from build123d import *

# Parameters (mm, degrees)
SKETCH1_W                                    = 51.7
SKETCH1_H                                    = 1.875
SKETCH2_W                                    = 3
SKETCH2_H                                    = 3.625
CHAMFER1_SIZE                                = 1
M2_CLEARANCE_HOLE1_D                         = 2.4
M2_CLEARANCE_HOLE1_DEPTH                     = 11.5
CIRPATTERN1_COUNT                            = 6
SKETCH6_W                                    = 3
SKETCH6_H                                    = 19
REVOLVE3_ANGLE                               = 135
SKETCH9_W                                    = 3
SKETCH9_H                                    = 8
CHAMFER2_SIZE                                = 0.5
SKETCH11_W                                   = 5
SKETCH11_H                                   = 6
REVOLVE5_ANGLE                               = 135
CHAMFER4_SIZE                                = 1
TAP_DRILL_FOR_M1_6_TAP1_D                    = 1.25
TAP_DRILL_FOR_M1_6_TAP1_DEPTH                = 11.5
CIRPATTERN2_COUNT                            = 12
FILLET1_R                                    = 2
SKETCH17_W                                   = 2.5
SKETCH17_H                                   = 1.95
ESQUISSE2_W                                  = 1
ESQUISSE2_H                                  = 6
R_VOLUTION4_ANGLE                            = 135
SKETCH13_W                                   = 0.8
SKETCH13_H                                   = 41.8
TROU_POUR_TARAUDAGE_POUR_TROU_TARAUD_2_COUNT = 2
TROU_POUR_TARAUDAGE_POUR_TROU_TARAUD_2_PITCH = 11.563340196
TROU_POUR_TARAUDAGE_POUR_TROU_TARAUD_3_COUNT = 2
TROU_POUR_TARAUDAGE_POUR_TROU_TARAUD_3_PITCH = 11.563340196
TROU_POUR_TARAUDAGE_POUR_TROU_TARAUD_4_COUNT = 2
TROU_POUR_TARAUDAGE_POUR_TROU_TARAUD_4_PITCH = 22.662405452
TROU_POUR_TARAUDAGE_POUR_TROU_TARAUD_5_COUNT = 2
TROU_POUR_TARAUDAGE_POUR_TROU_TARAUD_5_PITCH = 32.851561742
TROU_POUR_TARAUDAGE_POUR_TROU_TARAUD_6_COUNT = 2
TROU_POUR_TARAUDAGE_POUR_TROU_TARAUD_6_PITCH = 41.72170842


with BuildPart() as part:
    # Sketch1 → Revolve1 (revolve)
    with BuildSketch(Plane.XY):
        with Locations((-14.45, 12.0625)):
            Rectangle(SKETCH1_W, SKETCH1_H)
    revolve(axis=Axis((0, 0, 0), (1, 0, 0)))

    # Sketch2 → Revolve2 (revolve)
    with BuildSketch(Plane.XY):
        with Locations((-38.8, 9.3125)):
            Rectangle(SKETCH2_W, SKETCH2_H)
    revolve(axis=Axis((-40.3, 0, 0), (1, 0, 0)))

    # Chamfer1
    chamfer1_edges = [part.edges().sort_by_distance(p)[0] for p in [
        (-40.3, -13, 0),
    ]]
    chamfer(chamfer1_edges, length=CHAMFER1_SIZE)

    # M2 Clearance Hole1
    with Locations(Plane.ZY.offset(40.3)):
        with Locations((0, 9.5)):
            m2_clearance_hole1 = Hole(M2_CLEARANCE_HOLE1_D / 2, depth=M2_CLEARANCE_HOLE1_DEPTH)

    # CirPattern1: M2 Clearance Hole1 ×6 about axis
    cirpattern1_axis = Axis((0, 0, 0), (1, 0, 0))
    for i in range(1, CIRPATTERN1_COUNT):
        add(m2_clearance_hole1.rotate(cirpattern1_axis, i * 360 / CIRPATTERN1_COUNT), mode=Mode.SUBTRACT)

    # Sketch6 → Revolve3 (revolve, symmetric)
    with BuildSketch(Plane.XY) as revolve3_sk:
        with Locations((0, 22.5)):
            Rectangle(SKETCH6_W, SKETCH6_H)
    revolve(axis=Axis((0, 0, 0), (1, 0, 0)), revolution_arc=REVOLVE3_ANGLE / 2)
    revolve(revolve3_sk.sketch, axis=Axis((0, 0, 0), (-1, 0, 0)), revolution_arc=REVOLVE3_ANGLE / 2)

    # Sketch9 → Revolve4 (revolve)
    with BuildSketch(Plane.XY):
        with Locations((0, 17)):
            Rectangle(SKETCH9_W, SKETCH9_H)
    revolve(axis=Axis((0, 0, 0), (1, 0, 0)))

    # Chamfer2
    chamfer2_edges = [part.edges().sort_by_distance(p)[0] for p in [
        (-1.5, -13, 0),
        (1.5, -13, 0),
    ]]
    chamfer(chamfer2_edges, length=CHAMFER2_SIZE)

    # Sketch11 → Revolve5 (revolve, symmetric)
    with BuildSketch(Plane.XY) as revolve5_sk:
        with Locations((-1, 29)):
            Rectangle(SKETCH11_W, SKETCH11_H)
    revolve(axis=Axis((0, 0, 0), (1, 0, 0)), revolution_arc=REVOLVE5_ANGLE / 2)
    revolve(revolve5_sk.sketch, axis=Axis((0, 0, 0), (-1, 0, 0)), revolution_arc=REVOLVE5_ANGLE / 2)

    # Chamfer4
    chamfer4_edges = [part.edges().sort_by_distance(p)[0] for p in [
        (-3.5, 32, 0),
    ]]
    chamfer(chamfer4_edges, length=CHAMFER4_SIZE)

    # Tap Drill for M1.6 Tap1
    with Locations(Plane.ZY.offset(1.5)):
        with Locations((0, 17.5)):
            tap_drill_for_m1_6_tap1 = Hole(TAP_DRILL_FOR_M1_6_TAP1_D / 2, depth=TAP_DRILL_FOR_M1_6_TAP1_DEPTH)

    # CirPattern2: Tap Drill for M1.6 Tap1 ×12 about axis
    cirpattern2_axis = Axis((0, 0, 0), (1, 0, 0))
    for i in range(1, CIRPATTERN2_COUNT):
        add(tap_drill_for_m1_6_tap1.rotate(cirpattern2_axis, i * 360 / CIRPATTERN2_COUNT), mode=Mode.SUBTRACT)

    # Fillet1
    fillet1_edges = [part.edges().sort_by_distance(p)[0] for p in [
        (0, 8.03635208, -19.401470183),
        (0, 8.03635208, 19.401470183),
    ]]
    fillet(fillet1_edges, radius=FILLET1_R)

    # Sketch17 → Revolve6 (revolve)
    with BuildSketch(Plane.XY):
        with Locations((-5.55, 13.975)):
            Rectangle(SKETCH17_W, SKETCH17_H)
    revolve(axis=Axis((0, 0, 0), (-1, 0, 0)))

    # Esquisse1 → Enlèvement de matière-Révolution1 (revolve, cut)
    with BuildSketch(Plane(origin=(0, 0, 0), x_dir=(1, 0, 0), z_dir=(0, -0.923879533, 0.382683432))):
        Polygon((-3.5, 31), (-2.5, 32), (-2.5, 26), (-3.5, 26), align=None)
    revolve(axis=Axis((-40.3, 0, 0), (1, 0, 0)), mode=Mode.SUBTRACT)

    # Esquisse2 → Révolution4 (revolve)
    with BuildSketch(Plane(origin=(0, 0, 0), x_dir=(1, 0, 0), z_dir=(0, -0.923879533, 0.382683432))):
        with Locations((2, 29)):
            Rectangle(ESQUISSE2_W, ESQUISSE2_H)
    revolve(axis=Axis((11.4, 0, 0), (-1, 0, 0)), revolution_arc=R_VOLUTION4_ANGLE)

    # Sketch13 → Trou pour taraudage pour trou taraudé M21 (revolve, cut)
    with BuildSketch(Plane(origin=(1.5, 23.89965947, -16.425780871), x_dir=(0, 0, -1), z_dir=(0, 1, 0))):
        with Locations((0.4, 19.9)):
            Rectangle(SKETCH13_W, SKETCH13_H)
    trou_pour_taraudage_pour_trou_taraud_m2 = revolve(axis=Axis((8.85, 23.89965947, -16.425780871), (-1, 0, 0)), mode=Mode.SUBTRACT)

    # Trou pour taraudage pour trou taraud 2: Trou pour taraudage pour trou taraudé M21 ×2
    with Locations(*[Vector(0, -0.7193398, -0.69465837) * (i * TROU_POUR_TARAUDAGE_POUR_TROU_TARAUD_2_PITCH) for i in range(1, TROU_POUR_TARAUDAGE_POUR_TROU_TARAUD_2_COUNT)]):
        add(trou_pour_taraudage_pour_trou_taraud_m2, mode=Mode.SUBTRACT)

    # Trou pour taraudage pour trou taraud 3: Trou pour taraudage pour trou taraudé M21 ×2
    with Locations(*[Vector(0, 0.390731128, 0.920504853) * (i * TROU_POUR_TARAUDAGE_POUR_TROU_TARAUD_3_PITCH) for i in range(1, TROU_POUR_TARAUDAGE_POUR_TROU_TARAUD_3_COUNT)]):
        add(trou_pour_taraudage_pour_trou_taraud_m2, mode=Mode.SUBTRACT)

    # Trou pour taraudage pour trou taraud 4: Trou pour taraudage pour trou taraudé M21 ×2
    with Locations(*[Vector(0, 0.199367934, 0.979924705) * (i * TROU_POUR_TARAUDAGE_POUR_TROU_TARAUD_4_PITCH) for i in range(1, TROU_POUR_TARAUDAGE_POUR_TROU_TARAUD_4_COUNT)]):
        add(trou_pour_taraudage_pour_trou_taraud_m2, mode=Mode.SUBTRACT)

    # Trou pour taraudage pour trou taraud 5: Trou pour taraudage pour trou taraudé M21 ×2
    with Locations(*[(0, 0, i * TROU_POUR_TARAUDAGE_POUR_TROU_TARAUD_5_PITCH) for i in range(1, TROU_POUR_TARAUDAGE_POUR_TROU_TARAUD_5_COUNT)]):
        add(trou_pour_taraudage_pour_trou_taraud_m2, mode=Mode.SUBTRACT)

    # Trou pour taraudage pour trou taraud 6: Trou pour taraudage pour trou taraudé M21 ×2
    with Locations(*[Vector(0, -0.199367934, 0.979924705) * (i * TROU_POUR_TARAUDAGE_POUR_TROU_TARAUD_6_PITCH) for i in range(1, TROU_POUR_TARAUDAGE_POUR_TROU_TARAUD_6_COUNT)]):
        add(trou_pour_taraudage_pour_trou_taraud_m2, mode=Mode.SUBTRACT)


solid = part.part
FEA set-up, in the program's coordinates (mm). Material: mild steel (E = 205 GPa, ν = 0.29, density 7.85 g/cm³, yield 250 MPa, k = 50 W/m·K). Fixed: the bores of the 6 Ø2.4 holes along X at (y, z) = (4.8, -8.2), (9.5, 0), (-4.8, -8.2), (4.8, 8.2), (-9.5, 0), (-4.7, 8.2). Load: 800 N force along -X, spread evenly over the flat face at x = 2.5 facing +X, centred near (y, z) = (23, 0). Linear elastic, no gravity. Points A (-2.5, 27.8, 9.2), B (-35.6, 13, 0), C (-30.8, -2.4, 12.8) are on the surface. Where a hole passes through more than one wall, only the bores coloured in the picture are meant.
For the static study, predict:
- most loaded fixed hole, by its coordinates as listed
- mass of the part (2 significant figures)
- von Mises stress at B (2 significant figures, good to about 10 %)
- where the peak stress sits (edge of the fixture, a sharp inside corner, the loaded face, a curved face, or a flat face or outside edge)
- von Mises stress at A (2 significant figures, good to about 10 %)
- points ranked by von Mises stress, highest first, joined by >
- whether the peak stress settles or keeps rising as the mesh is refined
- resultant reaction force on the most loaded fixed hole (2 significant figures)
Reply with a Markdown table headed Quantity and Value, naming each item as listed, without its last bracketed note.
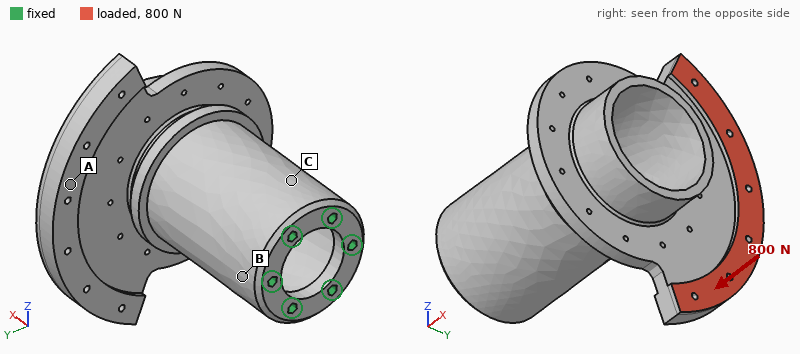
| Quantity | Value |
|---|---|
| most loaded fixed hole, by its coordinates as listed | (9.5, 0) |
| mass of the part | 110 g |
| von Mises stress at B | 30 MPa |
| where the peak stress sits | edge of the fixture |
| von Mises stress at A | 39 MPa |
| points ranked by von Mises stress, highest first, joined by > | A > B > C |
| whether the peak stress settles or keeps rising as the mesh is refined | keeps rising |
| resultant reaction force on the most loaded fixed hole | 610 N |
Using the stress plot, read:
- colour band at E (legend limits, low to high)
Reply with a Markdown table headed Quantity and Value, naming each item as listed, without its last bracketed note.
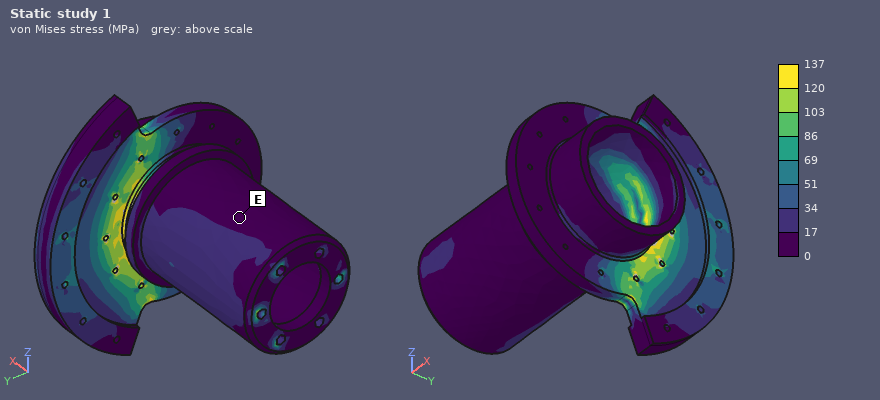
| Quantity | Value |
|---|---|
| colour band at E | 0 to 17 MPa |
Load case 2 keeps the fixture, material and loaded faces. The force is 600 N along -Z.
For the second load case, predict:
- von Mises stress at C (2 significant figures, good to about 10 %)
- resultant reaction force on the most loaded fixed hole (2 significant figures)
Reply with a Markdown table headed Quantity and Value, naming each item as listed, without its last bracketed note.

| Quantity | Value |
|---|---|
| von Mises stress at C | 27 MPa |
| resultant reaction force on the most loaded fixed hole | 680 N |
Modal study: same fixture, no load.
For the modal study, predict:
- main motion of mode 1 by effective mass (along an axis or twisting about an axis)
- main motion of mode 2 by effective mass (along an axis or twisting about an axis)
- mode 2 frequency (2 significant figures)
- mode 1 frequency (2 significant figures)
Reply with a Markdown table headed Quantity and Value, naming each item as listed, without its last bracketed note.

| Quantity | Value |
|---|---|
| main motion of mode 1 by effective mass | along Y |
| main motion of mode 2 by effective mass | along Z |
| mode 2 frequency | 3500 Hz |
| mode 1 frequency | 3300 Hz |
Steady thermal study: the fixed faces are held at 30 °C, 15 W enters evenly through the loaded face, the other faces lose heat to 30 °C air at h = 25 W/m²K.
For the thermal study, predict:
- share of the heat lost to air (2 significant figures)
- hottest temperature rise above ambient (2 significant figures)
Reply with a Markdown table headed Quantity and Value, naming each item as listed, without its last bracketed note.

| Quantity | Value |
|---|---|
| share of the heat lost to air | 61 % |
| hottest temperature rise above ambient | 71 K |
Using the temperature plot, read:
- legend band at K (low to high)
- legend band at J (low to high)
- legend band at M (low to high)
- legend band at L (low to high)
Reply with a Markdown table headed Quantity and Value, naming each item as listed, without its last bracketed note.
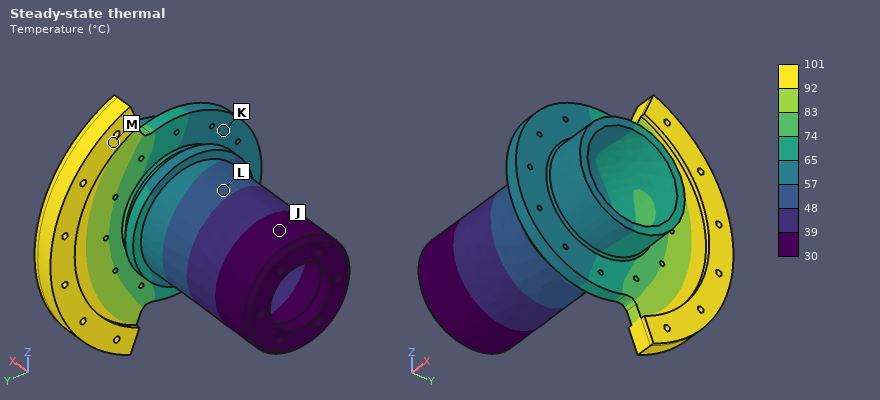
| Quantity | Value |
|---|---|
| legend band at K | 57 to 65 °C |
| legend band at J | 30 to 39 °C |
| legend band at M | 92 to 101 °C |
| legend band at L | 48 to 57 °C |
